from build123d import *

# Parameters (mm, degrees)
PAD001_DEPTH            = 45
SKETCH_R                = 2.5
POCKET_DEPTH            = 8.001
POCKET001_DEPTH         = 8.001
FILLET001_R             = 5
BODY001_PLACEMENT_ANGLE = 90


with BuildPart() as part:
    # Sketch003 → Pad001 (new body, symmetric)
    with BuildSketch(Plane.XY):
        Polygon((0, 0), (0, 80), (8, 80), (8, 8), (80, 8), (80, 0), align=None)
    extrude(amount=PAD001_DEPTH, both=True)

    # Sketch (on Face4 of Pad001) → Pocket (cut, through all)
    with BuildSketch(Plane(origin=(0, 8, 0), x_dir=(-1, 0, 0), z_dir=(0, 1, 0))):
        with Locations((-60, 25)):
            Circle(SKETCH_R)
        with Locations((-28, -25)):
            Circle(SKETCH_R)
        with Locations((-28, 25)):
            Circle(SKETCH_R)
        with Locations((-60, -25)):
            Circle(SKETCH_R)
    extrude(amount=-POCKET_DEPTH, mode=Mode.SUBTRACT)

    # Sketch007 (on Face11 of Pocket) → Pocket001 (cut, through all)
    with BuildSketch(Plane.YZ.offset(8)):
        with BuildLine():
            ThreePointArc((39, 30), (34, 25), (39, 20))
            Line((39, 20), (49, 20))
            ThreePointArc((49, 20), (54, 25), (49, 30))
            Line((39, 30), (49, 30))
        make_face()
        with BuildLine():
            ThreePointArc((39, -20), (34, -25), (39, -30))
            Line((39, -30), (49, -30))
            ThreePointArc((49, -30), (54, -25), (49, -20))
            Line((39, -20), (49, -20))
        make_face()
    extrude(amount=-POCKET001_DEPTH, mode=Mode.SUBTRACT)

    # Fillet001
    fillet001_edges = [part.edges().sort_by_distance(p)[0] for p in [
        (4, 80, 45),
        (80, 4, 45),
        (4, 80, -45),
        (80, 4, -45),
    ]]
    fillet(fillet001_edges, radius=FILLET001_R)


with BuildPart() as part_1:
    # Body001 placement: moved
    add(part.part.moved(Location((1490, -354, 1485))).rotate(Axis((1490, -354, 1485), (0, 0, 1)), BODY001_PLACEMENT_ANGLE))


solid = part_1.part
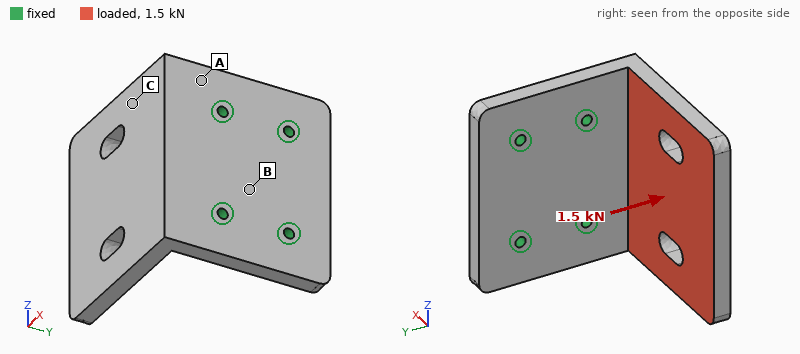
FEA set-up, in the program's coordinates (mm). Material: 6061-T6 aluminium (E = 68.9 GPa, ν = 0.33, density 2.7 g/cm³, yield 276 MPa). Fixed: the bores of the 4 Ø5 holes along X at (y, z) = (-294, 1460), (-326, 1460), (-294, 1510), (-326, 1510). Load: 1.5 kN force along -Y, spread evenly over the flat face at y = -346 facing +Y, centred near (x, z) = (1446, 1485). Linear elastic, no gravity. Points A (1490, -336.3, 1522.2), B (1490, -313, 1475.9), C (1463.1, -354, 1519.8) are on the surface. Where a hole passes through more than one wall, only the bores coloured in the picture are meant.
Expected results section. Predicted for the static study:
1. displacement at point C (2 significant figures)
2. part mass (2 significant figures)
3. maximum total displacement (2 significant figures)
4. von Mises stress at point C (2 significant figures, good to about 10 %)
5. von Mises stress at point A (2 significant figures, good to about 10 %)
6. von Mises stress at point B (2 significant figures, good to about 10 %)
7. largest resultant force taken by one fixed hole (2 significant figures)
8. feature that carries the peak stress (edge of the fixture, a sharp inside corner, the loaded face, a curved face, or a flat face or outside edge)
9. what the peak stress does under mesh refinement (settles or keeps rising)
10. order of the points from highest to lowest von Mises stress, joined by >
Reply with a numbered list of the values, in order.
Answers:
1. 0.19 mm
2. 290 g
3. 0.72 mm
4. 30 MPa
5. 55 MPa
6. 11 MPa
7. 730 N
8. edge of the fixture
9. keeps rising
10. A > C > B
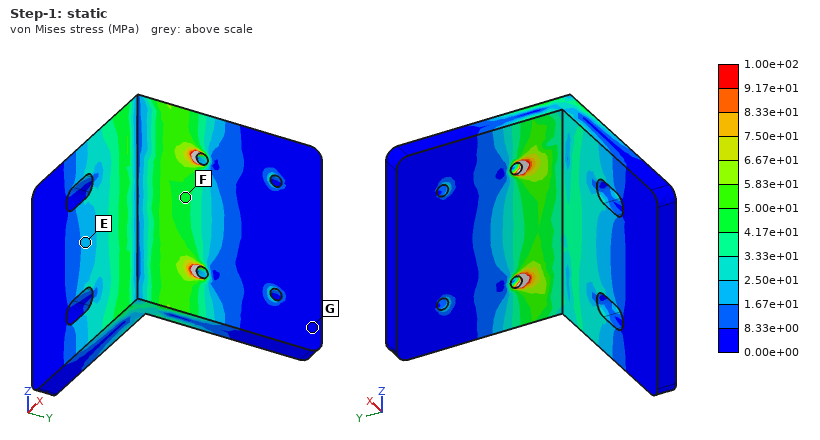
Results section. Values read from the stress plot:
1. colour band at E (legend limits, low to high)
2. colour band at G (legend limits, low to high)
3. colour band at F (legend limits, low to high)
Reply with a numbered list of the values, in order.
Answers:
1. 1.67e+01 to 2.50e+01 MPa
2. 0.00e+00 to 8.33e+00 MPa
3. 4.17e+01 to 5.00e+01 MPa
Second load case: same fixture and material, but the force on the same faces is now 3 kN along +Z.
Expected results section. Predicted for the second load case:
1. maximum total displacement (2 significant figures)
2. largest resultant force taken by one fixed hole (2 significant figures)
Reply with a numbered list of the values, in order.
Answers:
1. 0.25 mm
2. 2.9 kN
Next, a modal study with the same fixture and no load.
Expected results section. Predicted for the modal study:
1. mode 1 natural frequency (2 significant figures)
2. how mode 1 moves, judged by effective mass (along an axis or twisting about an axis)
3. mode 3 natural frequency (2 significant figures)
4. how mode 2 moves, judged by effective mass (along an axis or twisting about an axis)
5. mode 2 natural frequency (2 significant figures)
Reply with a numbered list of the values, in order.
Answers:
1. 770 Hz
2. along Y
3. 2400 Hz
4. along Z
5. 1700 Hz
